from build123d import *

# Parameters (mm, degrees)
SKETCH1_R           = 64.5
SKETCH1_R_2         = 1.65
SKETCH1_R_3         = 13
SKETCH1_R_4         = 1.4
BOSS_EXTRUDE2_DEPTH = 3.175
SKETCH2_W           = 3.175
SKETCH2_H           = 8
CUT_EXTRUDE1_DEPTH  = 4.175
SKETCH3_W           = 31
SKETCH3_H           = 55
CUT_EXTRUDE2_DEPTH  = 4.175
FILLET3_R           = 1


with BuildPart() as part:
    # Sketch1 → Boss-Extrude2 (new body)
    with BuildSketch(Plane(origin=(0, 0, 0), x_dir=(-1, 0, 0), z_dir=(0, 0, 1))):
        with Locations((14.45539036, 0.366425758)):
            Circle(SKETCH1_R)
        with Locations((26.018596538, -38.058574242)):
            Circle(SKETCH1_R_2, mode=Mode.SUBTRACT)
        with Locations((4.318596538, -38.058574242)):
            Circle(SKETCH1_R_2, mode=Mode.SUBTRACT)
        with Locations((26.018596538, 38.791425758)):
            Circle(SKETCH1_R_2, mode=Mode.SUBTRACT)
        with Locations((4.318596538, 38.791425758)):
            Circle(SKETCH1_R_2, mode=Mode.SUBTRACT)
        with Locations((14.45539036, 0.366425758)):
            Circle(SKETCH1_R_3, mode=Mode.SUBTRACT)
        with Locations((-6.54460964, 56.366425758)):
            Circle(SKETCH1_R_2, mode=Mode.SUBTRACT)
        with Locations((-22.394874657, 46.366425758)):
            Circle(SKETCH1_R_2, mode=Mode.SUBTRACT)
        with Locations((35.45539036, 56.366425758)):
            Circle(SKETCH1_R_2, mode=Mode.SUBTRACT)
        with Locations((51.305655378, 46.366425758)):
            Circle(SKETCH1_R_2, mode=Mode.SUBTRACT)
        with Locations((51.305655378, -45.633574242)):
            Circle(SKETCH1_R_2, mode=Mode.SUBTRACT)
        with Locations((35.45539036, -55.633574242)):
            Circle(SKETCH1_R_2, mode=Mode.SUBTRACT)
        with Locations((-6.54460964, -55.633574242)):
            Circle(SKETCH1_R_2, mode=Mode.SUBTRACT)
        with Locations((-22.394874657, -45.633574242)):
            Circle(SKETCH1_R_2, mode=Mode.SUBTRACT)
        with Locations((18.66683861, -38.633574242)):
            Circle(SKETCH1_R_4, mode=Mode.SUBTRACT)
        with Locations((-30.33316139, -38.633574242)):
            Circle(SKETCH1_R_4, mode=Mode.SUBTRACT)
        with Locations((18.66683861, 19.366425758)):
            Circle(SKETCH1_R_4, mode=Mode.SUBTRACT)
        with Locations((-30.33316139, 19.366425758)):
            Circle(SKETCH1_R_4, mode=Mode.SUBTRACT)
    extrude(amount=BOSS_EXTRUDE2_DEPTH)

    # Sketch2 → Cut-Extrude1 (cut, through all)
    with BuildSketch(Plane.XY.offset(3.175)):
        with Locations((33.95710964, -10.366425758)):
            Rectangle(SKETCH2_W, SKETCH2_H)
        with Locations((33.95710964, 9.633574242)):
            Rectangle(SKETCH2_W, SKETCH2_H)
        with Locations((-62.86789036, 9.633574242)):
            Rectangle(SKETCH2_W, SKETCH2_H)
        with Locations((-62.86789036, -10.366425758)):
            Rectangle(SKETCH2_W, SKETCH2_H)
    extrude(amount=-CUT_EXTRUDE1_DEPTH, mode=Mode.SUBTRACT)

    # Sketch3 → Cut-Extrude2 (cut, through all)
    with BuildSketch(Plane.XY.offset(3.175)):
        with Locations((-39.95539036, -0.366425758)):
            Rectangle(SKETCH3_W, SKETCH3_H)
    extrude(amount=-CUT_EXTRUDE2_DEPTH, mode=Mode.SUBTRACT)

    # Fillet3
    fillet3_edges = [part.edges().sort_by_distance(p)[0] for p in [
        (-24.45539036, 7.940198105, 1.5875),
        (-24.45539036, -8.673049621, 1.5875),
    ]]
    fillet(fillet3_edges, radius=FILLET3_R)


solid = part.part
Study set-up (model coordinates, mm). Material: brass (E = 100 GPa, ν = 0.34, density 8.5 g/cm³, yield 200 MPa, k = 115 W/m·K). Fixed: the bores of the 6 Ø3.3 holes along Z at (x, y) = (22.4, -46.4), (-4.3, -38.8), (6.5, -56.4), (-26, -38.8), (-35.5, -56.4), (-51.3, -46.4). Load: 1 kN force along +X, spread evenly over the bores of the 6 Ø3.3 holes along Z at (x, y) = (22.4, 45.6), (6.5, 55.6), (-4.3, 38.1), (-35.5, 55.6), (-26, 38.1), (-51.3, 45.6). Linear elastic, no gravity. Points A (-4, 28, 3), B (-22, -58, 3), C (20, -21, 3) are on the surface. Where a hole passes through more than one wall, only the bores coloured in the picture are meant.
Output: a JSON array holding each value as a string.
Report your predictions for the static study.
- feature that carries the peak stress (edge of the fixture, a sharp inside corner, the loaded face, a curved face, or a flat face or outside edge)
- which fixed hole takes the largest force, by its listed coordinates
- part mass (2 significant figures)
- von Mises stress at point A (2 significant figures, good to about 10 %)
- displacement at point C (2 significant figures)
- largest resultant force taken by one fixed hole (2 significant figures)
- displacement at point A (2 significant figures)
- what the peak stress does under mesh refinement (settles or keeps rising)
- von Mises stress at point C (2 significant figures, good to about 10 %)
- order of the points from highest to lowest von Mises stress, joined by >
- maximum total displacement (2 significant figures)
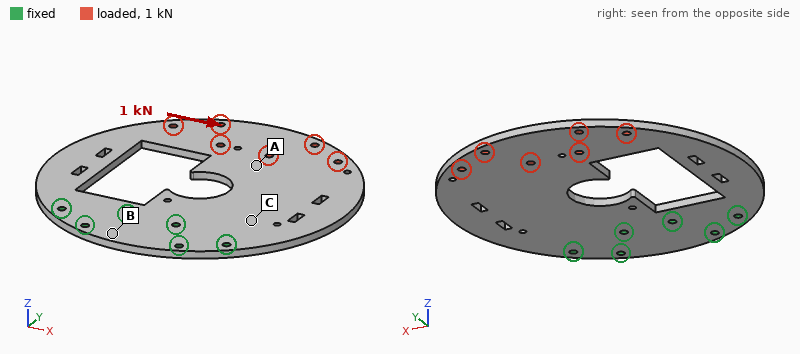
["edge of the fixture", "(22.4, -46.4)", "290 g", "9.5 MPa", "9.0 µm", "1.4 kN", "37 µm", "keeps rising", "15 MPa", "C > A > B", "52 µm"]
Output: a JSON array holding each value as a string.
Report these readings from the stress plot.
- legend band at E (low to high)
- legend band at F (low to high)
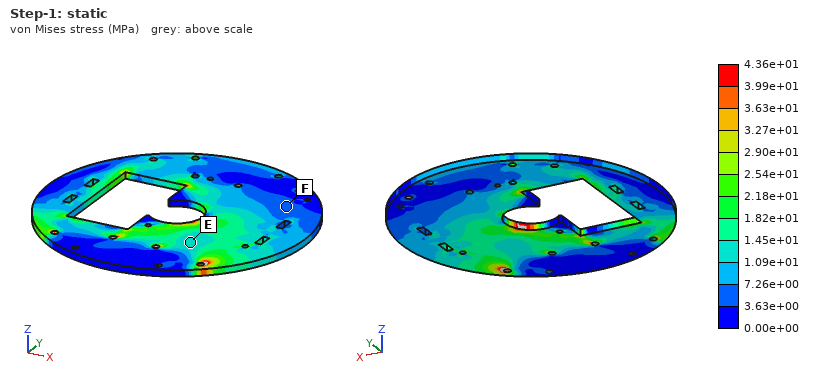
["1.09e+01 to 1.45e+01 MPa", "3.63e+00 to 7.26e+00 MPa"]
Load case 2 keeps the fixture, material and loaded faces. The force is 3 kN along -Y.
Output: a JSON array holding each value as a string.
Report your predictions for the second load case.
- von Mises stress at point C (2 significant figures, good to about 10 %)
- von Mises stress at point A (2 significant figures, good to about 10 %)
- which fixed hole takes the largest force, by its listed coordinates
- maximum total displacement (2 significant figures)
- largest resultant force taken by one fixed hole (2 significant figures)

["15 MPa", "22 MPa", "(-51.3, -46.4)", "41 µm", "1.2 kN"]
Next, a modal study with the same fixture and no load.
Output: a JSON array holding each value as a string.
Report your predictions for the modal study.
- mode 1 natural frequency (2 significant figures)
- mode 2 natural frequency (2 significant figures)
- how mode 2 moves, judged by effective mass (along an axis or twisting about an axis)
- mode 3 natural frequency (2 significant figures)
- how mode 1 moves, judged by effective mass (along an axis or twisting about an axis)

["150 Hz", "340 Hz", "twisting about Y", "750 Hz", "along Z"]
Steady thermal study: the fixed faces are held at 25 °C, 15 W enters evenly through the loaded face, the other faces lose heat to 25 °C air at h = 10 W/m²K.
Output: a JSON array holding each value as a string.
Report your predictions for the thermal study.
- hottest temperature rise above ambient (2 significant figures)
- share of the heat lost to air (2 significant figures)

["47 K", "32 %"]
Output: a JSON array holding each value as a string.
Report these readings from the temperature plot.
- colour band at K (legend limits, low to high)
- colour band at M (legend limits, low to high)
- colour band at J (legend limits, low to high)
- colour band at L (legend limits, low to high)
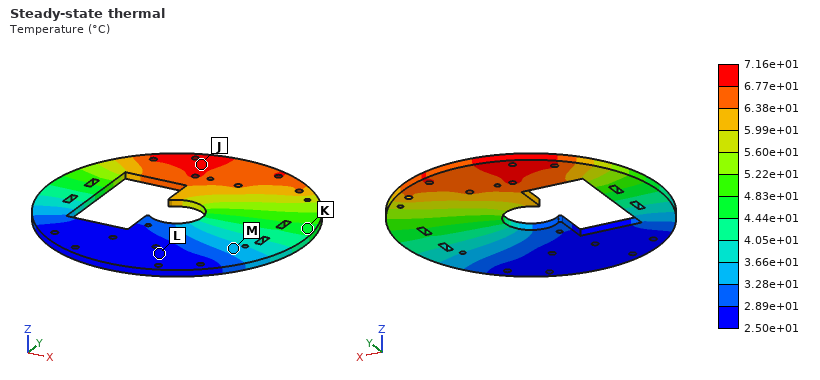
["4.44e+01 to 4.83e+01 °C", "3.28e+01 to 3.66e+01 °C", "6.77e+01 to 7.16e+01 °C", "2.50e+01 to 2.89e+01 °C"]
